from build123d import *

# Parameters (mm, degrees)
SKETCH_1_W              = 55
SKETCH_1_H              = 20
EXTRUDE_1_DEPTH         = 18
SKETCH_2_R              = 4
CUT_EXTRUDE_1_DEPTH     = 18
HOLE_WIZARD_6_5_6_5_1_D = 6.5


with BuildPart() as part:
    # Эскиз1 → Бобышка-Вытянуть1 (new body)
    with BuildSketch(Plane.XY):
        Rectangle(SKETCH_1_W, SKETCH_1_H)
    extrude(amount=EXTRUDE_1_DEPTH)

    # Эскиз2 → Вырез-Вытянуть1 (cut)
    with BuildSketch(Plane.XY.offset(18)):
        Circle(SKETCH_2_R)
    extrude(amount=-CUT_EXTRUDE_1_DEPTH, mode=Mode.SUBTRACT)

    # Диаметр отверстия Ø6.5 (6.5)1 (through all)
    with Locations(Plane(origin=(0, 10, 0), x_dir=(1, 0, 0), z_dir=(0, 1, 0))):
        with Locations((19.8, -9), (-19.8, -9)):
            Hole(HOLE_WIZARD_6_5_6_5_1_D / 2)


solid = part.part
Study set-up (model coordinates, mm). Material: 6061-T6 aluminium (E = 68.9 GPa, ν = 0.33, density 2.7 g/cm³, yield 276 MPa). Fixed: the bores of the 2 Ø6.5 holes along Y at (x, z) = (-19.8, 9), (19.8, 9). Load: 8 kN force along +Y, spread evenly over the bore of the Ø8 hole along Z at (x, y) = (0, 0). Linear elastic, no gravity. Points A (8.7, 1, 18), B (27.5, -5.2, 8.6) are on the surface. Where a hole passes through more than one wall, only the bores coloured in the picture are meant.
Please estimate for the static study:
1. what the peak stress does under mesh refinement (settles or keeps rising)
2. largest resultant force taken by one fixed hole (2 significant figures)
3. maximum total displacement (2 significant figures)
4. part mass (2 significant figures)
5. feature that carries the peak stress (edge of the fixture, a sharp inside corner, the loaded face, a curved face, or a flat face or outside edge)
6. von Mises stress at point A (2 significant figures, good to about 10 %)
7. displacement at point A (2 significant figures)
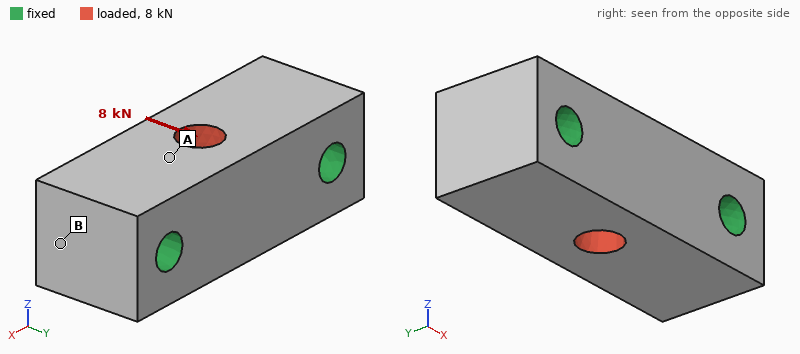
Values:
keeps rising
4.0 kN
12 µm
47 g
edge of the fixture
28 MPa
6.5 µm
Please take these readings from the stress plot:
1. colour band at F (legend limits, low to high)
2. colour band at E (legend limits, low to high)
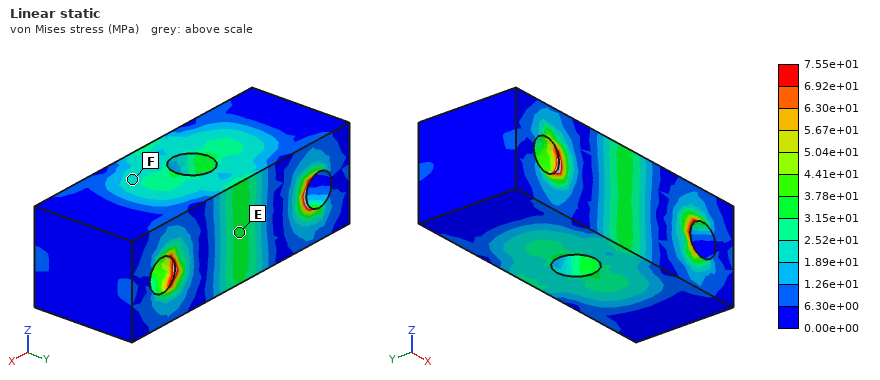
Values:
1.89e+01 to 2.52e+01 MPa
3.15e+01 to 3.78e+01 MPa
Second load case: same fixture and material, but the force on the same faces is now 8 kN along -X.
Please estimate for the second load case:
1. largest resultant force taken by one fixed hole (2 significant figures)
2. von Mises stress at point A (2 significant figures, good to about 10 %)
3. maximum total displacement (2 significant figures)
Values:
4.0 kN
15 MPa
3.7 µm
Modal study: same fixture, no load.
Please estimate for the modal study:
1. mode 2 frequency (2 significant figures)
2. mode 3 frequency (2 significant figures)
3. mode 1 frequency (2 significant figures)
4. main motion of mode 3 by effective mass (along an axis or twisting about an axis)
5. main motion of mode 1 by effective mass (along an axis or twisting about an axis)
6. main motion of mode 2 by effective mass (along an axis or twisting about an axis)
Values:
36 kHz
39 kHz
30 kHz
twisting about X
along Z
along Y
